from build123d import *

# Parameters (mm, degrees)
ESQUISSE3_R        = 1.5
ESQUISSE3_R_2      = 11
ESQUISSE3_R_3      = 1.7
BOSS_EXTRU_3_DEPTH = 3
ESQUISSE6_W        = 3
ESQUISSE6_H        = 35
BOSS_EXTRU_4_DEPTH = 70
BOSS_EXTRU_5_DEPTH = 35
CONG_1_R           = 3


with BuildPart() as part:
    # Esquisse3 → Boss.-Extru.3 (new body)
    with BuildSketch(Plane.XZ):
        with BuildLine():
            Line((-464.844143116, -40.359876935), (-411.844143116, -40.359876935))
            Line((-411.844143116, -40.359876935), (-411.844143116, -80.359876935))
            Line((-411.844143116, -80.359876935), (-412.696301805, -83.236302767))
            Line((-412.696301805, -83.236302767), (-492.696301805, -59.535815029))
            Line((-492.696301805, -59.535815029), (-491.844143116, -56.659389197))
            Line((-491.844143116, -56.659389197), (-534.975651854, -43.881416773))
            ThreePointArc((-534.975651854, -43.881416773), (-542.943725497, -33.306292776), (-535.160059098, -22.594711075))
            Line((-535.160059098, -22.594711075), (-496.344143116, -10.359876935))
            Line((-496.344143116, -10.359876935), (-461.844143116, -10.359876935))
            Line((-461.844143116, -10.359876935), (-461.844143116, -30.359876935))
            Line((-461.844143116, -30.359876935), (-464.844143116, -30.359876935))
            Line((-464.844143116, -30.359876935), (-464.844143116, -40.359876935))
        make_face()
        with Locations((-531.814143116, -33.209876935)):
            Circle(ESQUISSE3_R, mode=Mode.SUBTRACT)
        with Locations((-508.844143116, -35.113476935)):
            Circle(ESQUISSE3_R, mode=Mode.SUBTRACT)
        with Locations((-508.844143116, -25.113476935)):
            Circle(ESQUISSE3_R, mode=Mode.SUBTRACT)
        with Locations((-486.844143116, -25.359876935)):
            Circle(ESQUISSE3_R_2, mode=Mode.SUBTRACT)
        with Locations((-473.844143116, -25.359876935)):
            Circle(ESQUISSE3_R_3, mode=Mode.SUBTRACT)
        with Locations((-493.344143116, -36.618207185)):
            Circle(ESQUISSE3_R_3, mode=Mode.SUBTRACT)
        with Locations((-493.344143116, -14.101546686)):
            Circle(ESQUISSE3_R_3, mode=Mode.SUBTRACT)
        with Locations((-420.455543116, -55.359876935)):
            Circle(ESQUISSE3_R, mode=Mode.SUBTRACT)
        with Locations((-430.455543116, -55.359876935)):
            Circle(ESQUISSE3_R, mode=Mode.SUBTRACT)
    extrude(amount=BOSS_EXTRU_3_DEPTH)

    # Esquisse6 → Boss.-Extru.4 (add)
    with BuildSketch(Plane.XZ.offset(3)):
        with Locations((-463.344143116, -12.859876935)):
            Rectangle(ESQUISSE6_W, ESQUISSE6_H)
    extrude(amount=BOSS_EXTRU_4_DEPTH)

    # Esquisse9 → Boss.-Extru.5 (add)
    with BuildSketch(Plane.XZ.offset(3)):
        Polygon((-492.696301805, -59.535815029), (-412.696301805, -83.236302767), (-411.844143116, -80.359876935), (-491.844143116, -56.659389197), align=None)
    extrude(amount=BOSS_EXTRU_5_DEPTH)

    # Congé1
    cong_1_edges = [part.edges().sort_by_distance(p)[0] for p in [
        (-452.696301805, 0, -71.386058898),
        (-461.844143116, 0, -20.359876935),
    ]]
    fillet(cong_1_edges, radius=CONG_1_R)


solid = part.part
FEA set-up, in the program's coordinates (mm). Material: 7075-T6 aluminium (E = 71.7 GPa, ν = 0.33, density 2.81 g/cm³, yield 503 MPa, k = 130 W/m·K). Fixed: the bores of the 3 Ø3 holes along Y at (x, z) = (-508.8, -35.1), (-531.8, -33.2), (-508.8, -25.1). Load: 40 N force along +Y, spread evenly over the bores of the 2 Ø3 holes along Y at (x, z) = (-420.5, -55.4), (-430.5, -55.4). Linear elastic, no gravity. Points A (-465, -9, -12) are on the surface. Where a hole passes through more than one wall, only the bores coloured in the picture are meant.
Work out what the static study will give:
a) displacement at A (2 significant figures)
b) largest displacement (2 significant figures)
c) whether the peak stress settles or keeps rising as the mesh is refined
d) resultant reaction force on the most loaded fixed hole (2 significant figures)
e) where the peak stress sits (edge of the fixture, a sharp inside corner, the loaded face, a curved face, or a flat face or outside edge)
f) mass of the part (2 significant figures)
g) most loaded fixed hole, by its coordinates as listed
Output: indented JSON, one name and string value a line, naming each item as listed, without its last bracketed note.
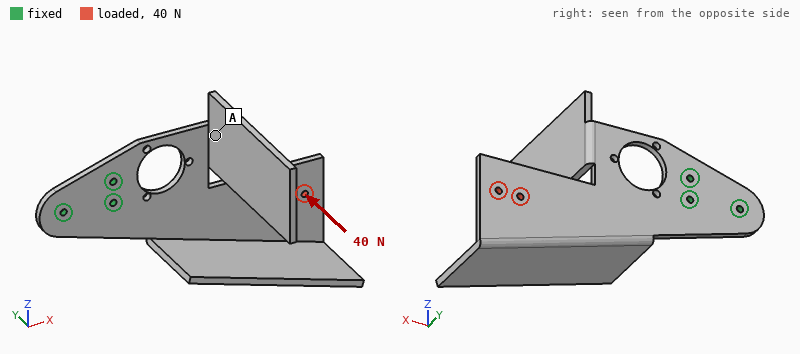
{
  "displacement at A": "0.41 mm",
  "largest displacement": "2.1 mm",
  "whether the peak stress settles or keeps rising as the mesh is refined": "keeps rising",
  "resultant reaction force on the most loaded fixed hole": "130 N",
  "where the peak stress sits": "a sharp inside corner",
  "mass of the part": "83 g",
  "most loaded fixed hole, by its coordinates as listed": "(-508.8, -35.1)"
}
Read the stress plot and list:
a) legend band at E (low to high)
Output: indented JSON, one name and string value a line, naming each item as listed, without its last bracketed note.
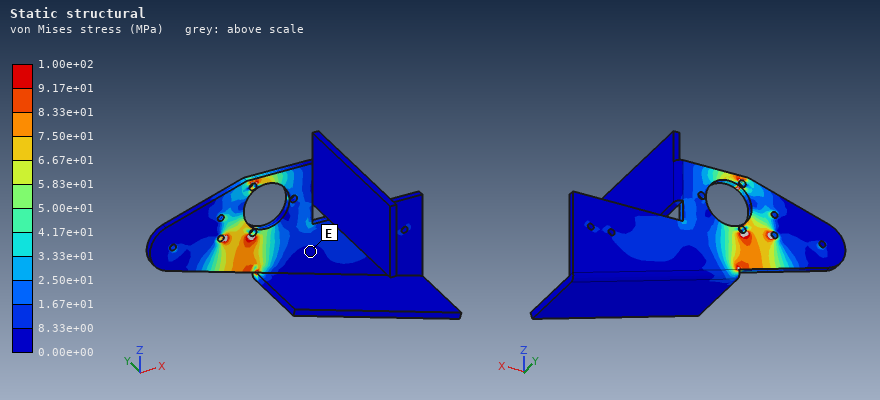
{
  "legend band at E": "0.00e+00 to 8.33e+00 MPa"
}
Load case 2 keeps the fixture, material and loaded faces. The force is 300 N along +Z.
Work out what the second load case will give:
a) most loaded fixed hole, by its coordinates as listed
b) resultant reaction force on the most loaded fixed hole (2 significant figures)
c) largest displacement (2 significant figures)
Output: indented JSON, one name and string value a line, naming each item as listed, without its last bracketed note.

{
  "most loaded fixed hole, by its coordinates as listed": "(-508.8, -25.1)",
  "resultant reaction force on the most loaded fixed hole": "960 N",
  "largest displacement": "0.28 mm"
}
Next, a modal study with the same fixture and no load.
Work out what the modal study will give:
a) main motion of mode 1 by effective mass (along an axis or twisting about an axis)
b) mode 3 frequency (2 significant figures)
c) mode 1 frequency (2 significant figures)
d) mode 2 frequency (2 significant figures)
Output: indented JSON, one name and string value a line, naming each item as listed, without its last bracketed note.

{
  "main motion of mode 1 by effective mass": "along Y",
  "mode 3 frequency": "360 Hz",
  "mode 1 frequency": "130 Hz",
  "mode 2 frequency": "200 Hz"
}
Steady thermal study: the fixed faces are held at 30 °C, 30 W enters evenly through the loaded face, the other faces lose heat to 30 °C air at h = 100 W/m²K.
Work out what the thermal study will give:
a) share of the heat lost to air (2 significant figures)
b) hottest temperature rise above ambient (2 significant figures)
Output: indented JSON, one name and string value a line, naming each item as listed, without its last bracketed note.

{
  "share of the heat lost to air": "92 %",
  "hottest temperature rise above ambient": "61 K"
}
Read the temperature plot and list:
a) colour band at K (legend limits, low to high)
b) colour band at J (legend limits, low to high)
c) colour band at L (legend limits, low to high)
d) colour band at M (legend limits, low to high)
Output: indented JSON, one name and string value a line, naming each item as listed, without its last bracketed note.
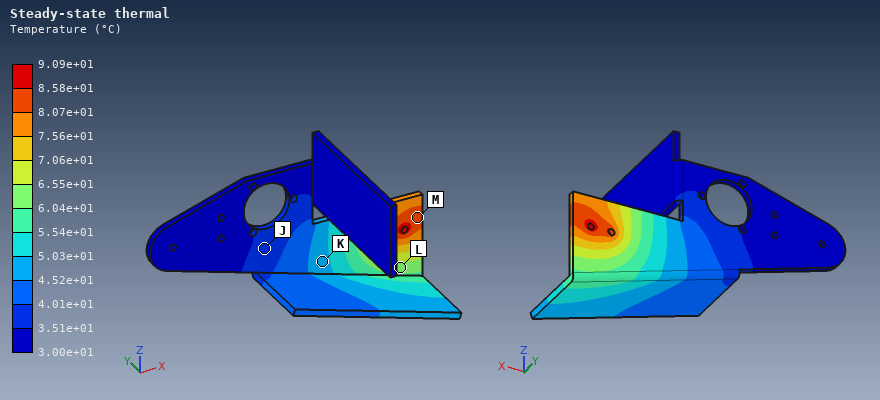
{
  "colour band at K": "4.52e+01 to 5.03e+01 °C",
  "colour band at J": "3.51e+01 to 4.01e+01 °C",
  "colour band at L": "6.04e+01 to 6.55e+01 °C",
  "colour band at M": "8.07e+01 to 8.58e+01 °C"
}
